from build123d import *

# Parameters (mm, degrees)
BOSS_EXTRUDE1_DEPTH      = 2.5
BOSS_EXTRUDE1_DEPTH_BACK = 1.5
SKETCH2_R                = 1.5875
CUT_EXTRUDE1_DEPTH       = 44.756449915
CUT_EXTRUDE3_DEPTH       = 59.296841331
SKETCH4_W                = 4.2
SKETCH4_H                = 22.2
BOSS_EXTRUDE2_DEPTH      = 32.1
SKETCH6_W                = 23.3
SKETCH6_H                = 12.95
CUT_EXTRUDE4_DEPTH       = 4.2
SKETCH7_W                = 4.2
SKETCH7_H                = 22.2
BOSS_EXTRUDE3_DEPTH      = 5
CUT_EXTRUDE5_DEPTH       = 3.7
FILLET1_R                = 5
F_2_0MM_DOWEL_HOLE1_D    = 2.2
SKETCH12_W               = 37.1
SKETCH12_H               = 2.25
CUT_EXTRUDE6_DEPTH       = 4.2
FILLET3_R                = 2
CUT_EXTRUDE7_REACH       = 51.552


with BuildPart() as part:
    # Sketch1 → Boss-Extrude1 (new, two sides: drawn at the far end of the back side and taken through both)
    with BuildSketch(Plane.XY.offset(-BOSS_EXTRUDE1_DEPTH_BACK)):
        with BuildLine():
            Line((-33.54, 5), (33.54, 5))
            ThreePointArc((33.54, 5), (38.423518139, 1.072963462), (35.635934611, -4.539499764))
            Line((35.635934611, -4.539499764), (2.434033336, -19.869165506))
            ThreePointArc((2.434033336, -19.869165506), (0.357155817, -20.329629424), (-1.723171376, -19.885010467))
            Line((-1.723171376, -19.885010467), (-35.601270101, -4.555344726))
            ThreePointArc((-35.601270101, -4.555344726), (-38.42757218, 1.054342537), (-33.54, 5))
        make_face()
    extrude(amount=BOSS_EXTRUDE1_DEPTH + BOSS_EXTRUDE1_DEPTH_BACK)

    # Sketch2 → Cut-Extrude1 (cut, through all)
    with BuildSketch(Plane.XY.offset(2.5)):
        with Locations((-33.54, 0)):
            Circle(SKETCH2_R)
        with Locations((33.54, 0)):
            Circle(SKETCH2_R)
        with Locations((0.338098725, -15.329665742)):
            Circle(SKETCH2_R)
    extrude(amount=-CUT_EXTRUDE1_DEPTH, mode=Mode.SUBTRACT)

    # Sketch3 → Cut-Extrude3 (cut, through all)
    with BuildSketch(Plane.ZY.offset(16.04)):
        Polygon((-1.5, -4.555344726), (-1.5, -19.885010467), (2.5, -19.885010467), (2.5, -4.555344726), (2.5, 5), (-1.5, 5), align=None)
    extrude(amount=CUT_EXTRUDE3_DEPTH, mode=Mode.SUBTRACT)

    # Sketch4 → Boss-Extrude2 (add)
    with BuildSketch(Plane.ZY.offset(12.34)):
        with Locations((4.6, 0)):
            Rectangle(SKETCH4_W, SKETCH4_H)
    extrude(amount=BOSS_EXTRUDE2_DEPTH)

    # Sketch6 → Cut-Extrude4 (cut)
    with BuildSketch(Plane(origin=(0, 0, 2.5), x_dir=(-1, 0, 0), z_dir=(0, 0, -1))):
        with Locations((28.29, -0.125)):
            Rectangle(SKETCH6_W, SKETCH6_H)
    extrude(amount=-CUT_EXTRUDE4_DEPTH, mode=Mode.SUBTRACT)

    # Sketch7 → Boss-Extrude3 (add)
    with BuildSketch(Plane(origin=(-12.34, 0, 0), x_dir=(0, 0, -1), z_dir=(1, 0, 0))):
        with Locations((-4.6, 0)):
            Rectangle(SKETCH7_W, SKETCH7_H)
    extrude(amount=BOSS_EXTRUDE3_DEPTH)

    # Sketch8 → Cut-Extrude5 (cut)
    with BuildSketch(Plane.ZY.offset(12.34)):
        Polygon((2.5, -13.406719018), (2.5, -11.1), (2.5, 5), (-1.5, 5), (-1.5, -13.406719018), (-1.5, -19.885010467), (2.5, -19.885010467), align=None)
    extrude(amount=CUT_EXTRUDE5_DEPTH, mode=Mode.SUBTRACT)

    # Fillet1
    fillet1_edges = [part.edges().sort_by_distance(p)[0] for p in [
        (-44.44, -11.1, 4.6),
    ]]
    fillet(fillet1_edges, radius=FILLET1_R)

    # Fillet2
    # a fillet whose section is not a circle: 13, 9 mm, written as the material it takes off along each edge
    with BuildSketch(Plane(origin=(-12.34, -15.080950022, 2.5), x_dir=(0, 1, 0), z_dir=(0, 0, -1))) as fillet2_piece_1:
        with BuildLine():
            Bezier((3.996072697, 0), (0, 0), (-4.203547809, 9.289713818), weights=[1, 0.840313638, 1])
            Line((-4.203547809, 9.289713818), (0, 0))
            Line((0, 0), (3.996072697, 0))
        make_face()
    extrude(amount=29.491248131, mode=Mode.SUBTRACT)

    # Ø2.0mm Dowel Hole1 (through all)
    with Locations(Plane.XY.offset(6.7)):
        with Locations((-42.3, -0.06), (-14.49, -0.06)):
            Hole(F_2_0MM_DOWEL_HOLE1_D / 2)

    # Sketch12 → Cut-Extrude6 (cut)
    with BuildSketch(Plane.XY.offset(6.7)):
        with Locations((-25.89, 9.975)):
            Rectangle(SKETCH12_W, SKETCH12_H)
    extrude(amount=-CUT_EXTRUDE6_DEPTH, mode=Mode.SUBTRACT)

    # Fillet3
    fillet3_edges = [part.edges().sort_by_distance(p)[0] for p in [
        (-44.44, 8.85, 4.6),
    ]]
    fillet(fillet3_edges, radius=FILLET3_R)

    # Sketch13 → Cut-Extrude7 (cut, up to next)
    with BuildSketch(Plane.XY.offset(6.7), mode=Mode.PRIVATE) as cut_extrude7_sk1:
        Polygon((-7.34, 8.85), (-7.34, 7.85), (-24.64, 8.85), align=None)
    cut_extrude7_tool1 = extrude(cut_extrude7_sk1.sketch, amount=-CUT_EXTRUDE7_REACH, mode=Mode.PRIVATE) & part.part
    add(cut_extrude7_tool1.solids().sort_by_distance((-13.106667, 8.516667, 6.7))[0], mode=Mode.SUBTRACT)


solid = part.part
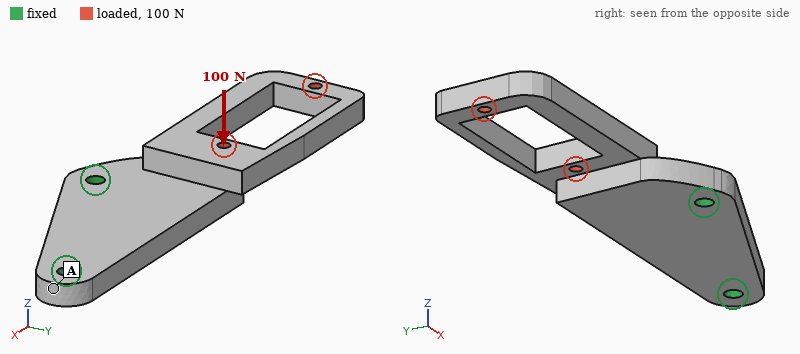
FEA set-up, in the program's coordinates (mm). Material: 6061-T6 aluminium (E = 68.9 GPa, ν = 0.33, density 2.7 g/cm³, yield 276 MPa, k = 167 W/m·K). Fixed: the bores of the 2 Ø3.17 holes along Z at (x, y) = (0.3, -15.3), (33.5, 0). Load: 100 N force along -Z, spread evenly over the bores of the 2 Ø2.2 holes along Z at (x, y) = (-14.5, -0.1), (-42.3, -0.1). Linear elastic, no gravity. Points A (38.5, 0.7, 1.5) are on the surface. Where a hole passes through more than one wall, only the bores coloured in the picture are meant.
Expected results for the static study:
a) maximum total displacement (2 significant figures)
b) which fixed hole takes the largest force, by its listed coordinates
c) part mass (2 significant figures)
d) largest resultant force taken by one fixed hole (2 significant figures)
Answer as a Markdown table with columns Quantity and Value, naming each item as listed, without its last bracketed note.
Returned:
| Quantity | Value |
|---|---|
| maximum total displacement | 0.41 mm |
| which fixed hole takes the largest force, by its listed coordinates | (0.3, -15.3) |
| part mass | 15 g |
| largest resultant force taken by one fixed hole | 130 N |
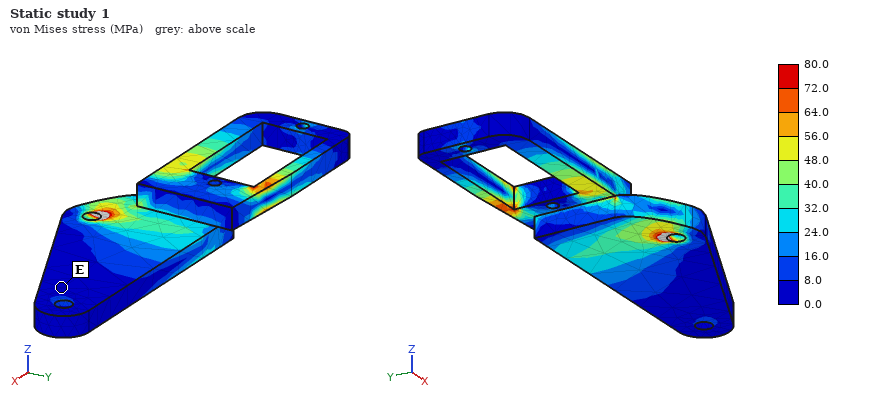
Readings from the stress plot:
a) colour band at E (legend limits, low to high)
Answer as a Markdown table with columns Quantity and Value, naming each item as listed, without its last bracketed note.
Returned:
| Quantity | Value |
|---|---|
| colour band at E | 0.0 to 8.0 MPa |
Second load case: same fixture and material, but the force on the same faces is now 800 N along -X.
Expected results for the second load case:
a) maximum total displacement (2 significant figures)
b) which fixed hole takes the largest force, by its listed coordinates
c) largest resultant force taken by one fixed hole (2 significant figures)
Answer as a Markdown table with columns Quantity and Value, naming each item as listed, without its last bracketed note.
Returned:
| Quantity | Value |
|---|---|
| maximum total displacement | 0.25 mm |
| which fixed hole takes the largest force, by its listed coordinates | (33.5, 0) |
| largest resultant force taken by one fixed hole | 530 N |
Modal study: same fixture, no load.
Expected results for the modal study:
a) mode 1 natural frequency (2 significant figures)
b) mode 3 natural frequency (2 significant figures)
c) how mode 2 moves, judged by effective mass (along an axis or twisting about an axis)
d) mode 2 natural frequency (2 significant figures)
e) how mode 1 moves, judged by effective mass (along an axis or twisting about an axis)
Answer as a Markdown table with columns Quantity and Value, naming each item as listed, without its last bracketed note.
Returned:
| Quantity | Value |
|---|---|
| mode 1 natural frequency | 1700 Hz |
| mode 3 natural frequency | 4700 Hz |
| how mode 2 moves, judged by effective mass | along Y |
| mode 2 natural frequency | 3600 Hz |
| how mode 1 moves, judged by effective mass | along Z |
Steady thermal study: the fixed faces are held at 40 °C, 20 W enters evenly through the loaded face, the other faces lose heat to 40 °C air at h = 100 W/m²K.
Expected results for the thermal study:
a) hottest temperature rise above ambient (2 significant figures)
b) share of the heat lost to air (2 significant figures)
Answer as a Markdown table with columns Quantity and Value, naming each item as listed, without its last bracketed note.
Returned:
| Quantity | Value |
|---|---|
| hottest temperature rise above ambient | 68 K |
| share of the heat lost to air | 35 % |
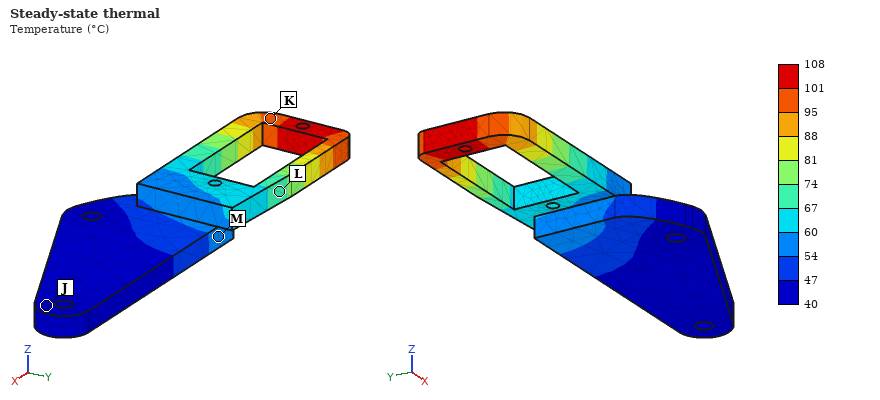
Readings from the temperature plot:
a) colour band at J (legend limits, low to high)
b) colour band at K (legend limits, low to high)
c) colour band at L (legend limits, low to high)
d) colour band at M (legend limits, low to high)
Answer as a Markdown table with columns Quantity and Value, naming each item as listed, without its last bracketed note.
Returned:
| Quantity | Value |
|---|---|
| colour band at J | 40 to 47 °C |
| colour band at K | 95 to 101 °C |
| colour band at L | 67 to 74 °C |
| colour band at M | 54 to 60 °C |
